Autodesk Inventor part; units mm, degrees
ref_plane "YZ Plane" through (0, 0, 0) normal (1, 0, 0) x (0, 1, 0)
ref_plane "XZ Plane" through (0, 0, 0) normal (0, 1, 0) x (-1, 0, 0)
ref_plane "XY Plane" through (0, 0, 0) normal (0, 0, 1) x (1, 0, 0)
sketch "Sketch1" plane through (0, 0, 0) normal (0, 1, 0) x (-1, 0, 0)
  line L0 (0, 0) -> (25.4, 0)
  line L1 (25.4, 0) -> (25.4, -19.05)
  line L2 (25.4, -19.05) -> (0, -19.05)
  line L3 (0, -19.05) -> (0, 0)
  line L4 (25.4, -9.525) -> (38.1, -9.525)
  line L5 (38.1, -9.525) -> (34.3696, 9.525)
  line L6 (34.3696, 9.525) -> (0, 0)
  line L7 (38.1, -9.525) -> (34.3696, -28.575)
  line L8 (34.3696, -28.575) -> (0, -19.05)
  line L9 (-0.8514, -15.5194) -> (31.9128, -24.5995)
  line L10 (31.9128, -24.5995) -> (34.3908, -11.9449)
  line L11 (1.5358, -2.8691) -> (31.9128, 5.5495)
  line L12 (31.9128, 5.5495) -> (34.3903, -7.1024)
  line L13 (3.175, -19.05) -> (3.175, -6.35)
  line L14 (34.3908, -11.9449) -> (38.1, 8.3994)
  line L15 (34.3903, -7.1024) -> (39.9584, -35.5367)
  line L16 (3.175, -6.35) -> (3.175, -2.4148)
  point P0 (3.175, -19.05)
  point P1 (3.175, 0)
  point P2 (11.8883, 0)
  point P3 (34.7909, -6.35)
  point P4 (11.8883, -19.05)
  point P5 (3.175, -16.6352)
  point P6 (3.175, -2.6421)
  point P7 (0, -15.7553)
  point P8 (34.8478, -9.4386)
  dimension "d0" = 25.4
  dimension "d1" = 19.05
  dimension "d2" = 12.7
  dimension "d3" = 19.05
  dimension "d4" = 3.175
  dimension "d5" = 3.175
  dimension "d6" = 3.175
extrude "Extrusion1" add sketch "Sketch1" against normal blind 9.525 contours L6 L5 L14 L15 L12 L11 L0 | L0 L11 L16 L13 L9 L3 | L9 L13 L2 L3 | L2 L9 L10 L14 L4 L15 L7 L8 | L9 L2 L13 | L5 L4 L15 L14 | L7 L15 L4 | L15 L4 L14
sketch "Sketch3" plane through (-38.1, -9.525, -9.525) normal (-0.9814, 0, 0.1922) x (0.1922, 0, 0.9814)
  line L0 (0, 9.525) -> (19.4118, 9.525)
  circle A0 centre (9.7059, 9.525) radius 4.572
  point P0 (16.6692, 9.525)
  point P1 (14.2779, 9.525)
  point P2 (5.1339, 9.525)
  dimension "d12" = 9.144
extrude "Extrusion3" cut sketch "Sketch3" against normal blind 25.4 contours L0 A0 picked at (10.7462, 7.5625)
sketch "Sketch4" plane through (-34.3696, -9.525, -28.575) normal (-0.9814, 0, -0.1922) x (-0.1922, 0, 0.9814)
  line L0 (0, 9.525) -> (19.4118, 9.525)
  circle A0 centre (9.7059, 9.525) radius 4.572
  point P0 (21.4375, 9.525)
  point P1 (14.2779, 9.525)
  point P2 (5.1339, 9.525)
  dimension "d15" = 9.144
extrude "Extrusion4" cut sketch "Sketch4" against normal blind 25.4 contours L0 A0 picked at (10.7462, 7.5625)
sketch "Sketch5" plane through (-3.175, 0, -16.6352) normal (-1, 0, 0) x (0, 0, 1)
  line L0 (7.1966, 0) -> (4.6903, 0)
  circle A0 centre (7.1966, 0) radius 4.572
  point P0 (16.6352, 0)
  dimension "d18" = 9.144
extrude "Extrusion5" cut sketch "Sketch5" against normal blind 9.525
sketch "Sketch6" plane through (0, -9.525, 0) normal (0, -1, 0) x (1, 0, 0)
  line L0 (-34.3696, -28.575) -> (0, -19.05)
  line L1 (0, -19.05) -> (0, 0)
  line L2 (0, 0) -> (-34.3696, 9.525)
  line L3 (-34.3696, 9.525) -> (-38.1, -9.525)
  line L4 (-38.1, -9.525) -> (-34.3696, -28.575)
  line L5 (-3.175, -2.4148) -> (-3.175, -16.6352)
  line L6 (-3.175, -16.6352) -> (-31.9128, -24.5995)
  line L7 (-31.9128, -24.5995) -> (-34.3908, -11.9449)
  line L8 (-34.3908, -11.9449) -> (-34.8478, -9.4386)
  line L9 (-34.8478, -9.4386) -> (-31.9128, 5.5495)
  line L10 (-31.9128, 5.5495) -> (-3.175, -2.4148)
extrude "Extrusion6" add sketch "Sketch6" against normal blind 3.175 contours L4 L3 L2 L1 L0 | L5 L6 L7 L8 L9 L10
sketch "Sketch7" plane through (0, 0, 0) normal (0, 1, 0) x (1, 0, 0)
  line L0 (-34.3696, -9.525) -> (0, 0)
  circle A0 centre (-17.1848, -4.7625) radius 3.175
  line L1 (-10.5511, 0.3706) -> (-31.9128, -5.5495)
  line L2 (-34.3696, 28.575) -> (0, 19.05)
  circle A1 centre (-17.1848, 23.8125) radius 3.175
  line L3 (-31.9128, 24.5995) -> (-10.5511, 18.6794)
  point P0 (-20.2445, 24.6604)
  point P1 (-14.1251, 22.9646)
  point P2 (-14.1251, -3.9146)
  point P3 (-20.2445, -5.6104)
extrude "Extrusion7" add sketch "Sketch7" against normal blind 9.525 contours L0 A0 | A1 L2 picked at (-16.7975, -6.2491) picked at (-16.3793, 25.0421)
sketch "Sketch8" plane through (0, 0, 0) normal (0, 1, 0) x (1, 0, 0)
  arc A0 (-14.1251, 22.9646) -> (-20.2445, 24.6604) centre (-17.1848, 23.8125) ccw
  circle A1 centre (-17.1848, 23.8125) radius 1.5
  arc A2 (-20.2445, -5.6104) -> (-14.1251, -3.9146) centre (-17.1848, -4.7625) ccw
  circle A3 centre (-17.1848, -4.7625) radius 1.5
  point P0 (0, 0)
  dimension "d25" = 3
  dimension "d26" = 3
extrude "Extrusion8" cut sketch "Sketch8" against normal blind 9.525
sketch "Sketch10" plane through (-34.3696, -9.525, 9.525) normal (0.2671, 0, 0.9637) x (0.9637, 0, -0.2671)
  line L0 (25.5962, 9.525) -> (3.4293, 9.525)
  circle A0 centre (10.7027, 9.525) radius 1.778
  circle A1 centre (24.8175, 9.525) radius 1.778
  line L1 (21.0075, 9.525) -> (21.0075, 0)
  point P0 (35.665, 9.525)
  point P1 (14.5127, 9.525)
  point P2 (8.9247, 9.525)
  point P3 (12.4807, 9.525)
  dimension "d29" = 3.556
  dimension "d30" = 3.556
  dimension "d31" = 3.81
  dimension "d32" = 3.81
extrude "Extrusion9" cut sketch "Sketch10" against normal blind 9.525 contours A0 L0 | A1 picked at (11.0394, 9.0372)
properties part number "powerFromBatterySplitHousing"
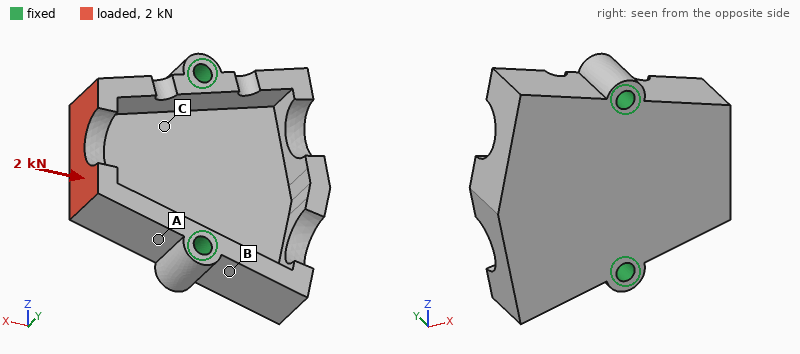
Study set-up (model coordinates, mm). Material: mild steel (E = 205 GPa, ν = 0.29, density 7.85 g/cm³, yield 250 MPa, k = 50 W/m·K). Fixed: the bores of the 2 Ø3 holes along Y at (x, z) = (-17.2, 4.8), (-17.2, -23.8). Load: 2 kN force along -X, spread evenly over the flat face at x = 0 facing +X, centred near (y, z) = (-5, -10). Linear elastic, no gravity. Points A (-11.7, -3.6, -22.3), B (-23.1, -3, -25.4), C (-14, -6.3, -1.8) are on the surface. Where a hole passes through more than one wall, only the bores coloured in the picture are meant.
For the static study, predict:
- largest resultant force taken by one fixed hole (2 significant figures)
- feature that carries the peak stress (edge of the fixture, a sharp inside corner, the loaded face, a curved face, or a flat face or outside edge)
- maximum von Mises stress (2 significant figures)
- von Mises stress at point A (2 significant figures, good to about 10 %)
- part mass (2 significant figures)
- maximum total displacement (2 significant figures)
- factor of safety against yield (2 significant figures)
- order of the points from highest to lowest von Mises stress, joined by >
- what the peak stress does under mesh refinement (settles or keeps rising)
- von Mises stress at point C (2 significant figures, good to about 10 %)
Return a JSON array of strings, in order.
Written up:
["1.0 kN", "a curved face", "96 MPa", "30 MPa", "43 g", "6.1 µm", "2.6", "A > C > B", "settles", "15 MPa"]
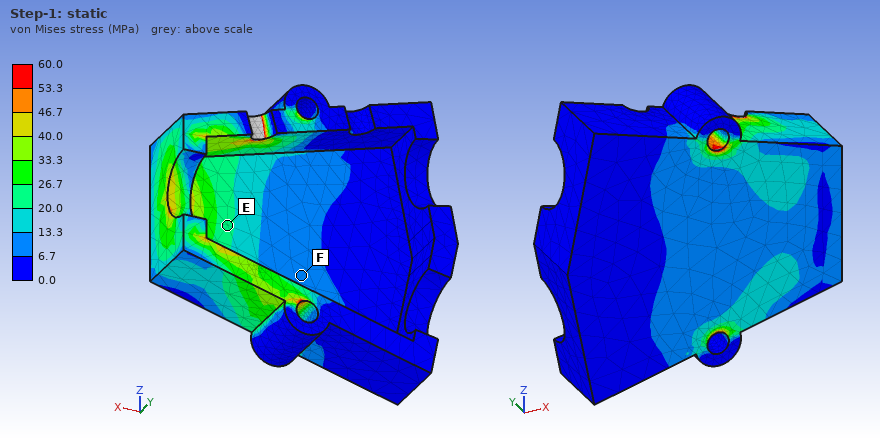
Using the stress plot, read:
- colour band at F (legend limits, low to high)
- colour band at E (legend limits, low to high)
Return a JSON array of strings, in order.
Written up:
["6.7 to 13.3 MPa", "20.0 to 26.7 MPa"]
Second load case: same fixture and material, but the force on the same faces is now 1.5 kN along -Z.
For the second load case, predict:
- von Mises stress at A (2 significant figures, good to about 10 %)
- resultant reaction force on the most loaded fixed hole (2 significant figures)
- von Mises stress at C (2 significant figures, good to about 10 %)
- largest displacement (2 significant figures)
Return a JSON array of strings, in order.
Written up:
["48 MPa", "1.2 kN", "33 MPa", "14 µm"]
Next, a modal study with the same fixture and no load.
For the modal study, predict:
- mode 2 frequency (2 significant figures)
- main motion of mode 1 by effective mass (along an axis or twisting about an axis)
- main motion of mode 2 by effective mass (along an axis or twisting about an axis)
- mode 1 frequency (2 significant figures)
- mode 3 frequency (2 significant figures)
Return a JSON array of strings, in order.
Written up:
["15 kHz", "along Y", "along Y", "9400 Hz", "17 kHz"]
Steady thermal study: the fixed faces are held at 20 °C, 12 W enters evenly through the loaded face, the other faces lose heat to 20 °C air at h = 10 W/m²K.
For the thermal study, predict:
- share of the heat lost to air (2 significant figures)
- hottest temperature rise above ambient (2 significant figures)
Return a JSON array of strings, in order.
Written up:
["3.3 %", "42 K"]
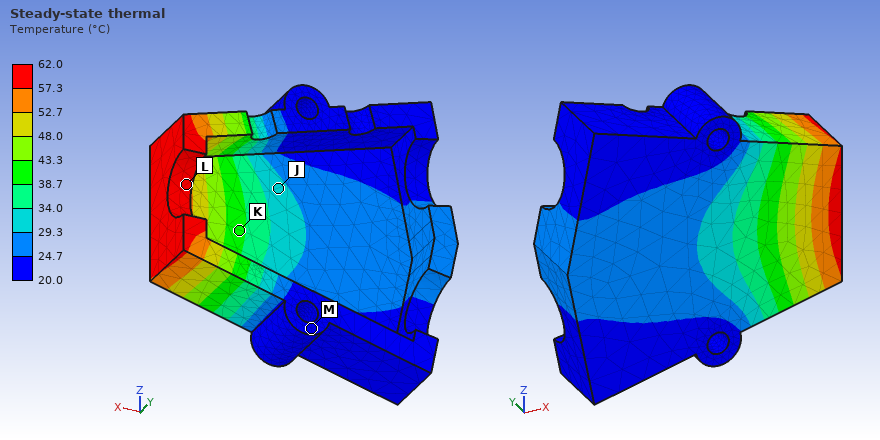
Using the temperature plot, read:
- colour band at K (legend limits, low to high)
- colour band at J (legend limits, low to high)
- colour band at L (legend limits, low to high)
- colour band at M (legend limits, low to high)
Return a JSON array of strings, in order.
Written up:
["38.7 to 43.3 °C", "29.3 to 34.0 °C", "57.3 to 62.0 °C", "20.0 to 24.7 °C"]
